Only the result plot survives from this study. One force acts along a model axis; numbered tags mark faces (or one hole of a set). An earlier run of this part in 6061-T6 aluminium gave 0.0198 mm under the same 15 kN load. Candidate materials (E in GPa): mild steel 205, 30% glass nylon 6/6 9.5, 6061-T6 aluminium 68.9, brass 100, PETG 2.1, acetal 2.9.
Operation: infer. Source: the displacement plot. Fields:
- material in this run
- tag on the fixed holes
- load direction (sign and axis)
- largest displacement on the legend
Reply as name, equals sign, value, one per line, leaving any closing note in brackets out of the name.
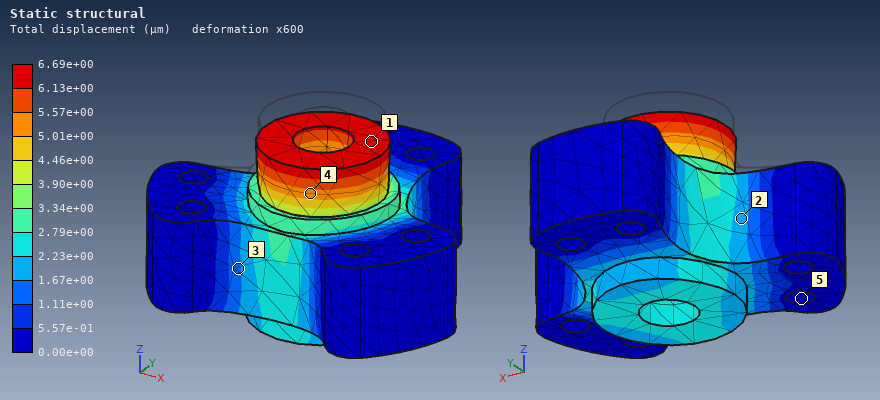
material in this run = mild steel
tag on the fixed holes = 5
load direction = -Z
largest displacement on the legend = 6.69e+00 µm
